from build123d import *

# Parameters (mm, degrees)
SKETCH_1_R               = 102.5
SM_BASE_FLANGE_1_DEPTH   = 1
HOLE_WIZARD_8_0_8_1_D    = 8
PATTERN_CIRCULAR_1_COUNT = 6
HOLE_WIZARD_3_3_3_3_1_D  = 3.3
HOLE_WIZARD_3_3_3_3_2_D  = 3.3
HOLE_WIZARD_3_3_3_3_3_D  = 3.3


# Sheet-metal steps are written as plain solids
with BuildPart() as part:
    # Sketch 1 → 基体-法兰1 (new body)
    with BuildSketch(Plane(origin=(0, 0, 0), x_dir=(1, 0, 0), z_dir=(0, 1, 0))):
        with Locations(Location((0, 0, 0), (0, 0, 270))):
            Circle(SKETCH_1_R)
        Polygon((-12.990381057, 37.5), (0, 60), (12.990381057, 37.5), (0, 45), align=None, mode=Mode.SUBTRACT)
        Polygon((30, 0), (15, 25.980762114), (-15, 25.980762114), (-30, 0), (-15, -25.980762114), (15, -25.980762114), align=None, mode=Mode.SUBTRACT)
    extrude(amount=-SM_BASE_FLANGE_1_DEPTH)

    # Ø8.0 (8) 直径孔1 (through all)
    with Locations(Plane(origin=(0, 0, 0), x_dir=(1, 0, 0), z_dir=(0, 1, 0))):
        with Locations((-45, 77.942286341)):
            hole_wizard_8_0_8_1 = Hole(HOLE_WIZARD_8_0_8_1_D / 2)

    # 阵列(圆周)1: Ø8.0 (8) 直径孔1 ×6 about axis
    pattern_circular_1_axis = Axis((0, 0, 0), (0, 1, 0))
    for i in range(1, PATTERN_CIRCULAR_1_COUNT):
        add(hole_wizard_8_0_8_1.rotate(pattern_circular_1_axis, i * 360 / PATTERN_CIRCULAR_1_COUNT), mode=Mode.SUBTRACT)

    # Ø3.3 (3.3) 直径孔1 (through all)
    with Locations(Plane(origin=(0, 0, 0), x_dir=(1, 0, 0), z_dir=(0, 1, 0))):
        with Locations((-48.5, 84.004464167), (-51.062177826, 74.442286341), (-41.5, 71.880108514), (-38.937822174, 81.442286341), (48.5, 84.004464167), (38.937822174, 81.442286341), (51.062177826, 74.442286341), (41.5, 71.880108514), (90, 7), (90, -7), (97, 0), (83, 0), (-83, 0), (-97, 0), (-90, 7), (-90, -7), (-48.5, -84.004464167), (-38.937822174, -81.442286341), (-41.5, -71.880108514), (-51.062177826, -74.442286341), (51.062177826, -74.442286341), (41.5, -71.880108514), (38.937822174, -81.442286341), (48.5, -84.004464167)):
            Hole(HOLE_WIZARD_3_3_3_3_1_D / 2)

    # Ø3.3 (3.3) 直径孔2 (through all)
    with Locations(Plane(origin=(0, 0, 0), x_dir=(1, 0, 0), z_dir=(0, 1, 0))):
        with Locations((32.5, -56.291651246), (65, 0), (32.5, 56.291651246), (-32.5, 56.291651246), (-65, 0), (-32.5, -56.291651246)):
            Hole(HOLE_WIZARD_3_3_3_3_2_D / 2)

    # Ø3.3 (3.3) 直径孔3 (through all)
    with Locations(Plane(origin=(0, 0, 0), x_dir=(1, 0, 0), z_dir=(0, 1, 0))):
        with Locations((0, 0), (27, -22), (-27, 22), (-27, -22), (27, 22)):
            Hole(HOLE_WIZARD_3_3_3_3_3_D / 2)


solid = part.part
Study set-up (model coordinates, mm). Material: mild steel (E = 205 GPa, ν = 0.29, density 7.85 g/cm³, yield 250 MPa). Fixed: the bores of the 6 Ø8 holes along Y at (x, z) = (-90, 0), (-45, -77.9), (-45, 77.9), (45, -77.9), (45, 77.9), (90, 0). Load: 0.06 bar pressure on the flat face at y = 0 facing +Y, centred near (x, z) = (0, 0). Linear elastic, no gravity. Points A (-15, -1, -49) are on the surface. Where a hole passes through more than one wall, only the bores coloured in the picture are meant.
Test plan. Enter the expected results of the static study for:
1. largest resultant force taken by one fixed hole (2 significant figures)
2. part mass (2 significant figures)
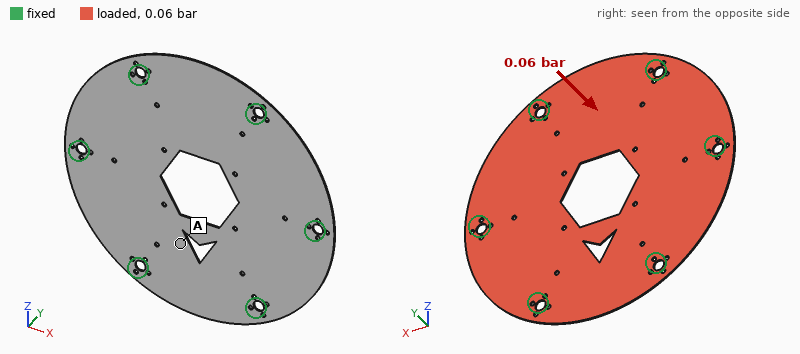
30 N
230 g
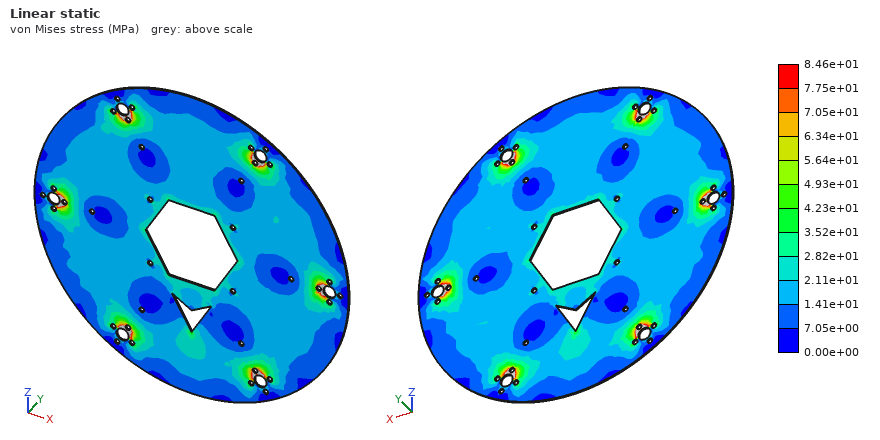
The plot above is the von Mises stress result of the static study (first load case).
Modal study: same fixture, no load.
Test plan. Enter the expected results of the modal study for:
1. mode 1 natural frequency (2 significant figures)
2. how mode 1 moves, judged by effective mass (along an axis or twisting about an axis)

290 Hz
along Y
